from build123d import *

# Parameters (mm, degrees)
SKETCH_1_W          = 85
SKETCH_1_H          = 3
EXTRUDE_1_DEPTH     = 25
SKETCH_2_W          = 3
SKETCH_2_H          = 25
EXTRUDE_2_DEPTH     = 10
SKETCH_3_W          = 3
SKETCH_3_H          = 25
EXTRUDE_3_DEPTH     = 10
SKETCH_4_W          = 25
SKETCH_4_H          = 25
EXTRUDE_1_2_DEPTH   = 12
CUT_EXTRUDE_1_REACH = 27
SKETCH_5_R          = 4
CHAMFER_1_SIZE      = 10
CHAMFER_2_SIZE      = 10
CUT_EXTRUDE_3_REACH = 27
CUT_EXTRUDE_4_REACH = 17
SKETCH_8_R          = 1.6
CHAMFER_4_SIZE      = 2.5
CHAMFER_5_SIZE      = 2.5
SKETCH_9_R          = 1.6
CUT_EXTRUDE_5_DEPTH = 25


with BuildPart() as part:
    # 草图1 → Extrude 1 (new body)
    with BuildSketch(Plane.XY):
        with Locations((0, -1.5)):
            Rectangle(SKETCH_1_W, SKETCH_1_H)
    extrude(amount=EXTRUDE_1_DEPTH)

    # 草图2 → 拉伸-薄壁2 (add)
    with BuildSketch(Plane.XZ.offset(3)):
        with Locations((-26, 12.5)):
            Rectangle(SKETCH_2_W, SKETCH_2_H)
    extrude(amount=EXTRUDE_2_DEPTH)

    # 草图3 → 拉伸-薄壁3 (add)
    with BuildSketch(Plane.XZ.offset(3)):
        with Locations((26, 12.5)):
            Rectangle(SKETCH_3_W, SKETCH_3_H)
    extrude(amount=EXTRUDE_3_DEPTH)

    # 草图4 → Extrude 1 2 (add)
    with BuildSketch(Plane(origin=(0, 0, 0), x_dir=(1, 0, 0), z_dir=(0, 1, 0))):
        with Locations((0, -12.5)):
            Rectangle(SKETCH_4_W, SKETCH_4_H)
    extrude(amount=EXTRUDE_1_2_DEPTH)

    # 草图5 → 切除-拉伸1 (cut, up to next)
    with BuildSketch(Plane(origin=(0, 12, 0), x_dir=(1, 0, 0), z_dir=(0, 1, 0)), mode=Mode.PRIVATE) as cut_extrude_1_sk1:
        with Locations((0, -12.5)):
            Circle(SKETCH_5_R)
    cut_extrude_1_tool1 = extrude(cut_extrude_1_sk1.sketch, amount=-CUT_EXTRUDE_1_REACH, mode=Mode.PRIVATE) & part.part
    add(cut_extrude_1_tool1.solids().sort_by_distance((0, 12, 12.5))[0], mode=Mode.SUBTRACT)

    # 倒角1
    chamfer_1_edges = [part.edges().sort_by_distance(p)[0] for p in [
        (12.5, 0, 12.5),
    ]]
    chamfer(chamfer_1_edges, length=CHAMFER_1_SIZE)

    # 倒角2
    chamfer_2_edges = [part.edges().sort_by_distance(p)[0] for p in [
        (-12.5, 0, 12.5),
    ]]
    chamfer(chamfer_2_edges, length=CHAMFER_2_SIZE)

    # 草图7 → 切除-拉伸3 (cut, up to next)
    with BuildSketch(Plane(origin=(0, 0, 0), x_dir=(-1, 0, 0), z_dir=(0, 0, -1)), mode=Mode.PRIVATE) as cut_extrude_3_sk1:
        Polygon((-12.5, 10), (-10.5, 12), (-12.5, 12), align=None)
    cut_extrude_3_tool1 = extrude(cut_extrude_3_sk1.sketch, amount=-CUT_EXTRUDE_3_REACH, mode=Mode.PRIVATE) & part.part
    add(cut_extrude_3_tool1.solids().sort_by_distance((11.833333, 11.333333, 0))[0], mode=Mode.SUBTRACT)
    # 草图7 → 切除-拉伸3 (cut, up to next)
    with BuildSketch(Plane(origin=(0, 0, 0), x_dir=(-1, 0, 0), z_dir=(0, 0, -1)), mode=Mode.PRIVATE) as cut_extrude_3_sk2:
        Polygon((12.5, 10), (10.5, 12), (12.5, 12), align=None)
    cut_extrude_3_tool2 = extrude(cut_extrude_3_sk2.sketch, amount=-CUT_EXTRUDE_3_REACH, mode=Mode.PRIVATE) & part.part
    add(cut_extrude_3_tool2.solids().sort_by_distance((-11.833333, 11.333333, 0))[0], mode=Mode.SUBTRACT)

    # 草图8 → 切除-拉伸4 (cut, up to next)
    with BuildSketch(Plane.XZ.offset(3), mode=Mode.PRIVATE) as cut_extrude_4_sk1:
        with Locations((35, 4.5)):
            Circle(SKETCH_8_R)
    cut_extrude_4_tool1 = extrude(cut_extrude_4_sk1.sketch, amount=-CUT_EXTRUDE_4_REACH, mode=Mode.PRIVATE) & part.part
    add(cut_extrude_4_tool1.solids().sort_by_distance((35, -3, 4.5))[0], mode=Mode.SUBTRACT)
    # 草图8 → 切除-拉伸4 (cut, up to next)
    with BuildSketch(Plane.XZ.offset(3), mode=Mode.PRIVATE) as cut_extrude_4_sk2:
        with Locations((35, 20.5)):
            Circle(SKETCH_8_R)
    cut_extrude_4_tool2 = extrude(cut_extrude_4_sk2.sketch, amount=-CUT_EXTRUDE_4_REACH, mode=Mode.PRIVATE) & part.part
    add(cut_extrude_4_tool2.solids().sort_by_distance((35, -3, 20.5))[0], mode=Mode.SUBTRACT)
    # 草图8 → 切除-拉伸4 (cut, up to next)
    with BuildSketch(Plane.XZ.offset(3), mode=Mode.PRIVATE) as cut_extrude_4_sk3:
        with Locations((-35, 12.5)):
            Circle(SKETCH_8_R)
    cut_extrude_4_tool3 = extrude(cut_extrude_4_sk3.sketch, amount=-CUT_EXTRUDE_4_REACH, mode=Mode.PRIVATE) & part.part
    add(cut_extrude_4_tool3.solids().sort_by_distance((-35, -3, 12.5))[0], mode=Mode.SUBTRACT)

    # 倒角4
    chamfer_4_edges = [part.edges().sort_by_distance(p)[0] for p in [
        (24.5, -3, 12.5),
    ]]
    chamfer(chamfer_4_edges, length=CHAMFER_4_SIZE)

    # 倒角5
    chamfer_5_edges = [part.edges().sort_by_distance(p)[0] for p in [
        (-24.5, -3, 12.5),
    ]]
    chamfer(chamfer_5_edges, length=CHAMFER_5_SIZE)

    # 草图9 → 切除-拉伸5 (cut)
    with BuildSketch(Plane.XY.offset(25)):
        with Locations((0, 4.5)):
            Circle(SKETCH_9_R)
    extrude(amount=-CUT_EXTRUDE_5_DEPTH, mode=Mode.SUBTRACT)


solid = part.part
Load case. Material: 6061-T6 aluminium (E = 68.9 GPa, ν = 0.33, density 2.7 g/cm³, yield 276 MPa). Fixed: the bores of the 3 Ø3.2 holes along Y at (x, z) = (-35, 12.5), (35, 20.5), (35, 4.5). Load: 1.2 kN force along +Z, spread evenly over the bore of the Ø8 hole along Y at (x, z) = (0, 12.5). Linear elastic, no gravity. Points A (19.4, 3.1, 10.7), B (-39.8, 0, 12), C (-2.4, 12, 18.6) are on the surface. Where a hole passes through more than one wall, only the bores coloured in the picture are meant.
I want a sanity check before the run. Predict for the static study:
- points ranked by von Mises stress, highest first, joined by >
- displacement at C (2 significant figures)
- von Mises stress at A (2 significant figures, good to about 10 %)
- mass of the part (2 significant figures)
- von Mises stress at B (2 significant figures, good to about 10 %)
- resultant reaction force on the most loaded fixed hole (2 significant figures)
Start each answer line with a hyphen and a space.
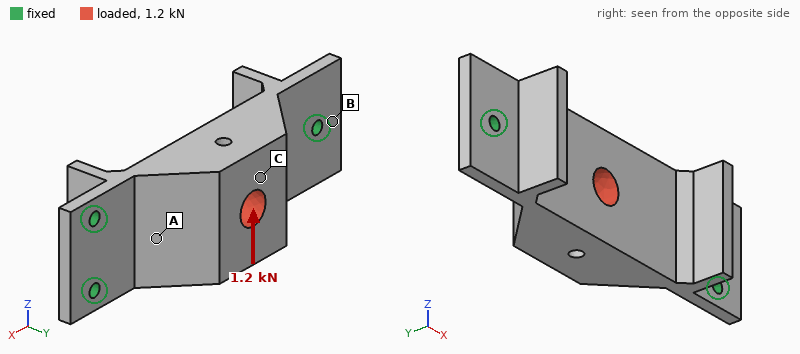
- A > B > C
- 68 µm
- 30 MPa
- 46 g
- 14 MPa
- 790 N
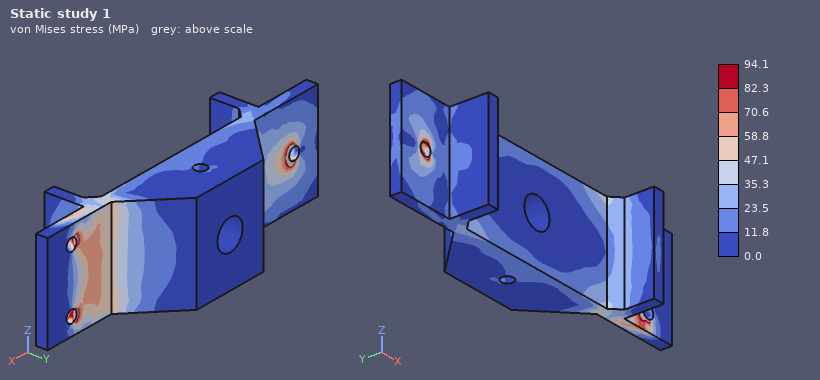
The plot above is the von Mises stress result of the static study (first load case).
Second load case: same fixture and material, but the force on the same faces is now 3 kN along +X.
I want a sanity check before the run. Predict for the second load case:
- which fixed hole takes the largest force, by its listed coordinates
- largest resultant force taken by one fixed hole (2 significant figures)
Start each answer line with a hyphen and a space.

- (-35, 12.5)
- 1.4 kN
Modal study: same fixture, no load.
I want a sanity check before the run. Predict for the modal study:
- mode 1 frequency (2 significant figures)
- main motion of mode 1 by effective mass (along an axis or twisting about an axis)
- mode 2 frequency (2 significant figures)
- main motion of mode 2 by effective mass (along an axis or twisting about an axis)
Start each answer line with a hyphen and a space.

- 3700 Hz
- along Z
- 4000 Hz
- along Y
